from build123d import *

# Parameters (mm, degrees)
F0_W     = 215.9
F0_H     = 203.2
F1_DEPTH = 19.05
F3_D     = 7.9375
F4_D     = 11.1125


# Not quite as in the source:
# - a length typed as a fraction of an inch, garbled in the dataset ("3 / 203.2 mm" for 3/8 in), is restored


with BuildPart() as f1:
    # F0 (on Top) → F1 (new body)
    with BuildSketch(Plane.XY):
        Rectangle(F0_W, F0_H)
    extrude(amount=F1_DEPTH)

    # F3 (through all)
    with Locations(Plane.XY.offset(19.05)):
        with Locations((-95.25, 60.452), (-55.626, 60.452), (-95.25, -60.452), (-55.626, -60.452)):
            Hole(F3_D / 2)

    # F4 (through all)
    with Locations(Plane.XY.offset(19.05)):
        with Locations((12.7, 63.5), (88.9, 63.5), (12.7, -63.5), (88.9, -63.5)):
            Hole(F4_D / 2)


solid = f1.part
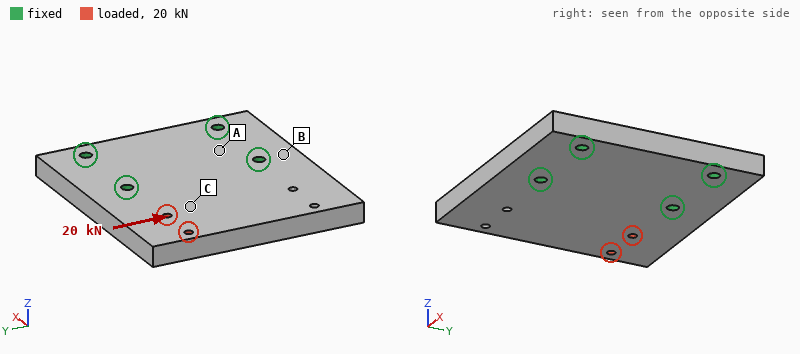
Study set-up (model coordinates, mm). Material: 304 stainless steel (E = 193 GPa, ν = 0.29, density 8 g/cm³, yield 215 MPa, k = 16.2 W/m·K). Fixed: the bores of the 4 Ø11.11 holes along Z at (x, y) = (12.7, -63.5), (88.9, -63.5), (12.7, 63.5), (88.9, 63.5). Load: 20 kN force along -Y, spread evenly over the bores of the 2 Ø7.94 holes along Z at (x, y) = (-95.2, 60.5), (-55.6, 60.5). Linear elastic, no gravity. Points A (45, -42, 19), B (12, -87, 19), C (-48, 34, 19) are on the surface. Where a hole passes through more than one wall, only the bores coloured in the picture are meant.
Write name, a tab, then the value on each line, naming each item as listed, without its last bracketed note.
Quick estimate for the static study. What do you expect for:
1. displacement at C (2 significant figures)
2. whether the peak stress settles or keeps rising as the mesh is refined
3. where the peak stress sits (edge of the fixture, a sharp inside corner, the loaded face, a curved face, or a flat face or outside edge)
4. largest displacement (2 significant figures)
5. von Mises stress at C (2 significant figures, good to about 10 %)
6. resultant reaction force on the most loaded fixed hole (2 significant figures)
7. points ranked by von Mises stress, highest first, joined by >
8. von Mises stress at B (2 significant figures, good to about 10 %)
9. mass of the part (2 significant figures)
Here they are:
displacement at C	8.3 µm
whether the peak stress settles or keeps rising as the mesh is refined	keeps rising
where the peak stress sits	edge of the fixture
largest displacement	18 µm
von Mises stress at C	15 MPa
resultant reaction force on the most loaded fixed hole	15 kN
points ranked by von Mises stress, highest first, joined by >	C > B > A
von Mises stress at B	8.4 MPa
mass of the part	6.6 kg
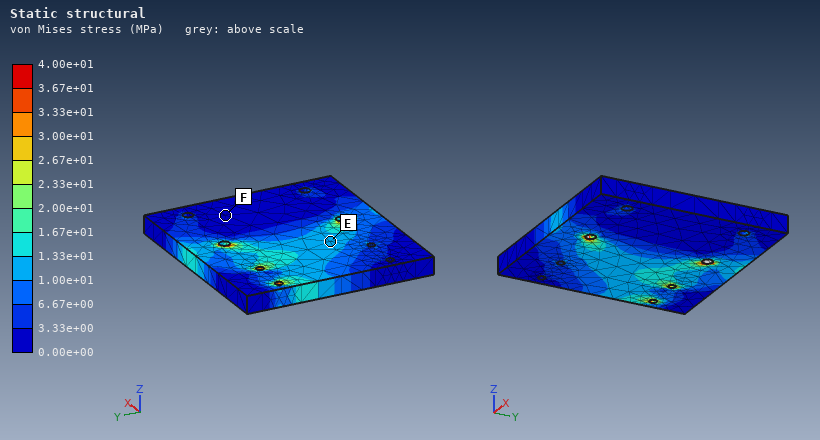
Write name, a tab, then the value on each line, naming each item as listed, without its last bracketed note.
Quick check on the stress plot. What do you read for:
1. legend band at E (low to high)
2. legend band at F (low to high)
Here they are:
legend band at E	1.00e+01 to 1.33e+01 MPa
legend band at F	0.00e+00 to 3.33e+00 MPa
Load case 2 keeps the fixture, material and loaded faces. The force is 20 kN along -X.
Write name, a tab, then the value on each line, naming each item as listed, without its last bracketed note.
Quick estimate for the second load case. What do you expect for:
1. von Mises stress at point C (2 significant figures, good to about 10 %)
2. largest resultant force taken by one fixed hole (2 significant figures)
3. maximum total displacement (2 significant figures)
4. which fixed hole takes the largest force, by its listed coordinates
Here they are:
von Mises stress at point C	8.2 MPa
largest resultant force taken by one fixed hole	15 kN
maximum total displacement	10.0 µm
which fixed hole takes the largest force, by its listed coordinates	(12.7, 63.5)
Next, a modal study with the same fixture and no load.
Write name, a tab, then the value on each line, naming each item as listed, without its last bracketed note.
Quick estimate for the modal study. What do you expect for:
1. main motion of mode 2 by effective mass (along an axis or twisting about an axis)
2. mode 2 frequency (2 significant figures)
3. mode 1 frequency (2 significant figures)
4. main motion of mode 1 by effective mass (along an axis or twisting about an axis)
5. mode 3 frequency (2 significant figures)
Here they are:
main motion of mode 2 by effective mass	twisting about X
mode 2 frequency	1600 Hz
mode 1 frequency	920 Hz
main motion of mode 1 by effective mass	along Z
mode 3 frequency	3100 Hz
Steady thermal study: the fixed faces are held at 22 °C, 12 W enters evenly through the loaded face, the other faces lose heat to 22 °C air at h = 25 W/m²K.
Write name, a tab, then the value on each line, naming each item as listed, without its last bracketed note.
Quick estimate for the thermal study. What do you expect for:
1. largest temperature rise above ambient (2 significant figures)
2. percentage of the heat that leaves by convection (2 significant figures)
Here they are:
largest temperature rise above ambient	21 K
percentage of the heat that leaves by convection	68 %
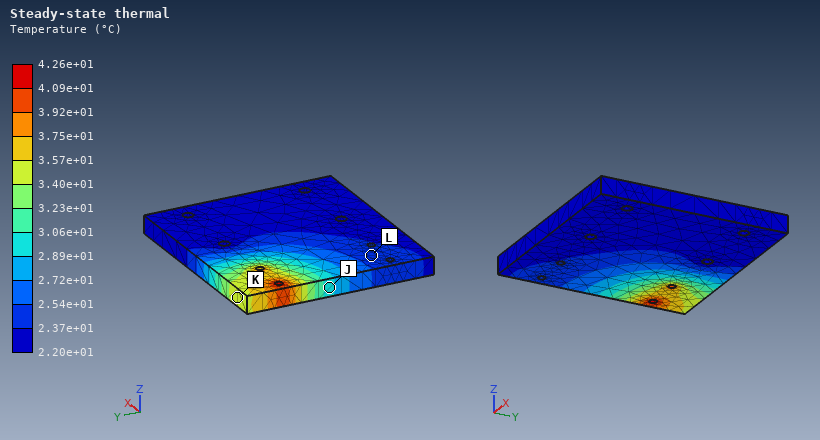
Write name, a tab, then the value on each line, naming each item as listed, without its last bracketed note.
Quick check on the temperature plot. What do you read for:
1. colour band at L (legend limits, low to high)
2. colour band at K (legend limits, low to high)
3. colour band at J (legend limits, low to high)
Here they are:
colour band at L	2.37e+01 to 2.54e+01 °C
colour band at K	3.40e+01 to 3.57e+01 °C
colour band at J	2.89e+01 to 3.06e+01 °C
